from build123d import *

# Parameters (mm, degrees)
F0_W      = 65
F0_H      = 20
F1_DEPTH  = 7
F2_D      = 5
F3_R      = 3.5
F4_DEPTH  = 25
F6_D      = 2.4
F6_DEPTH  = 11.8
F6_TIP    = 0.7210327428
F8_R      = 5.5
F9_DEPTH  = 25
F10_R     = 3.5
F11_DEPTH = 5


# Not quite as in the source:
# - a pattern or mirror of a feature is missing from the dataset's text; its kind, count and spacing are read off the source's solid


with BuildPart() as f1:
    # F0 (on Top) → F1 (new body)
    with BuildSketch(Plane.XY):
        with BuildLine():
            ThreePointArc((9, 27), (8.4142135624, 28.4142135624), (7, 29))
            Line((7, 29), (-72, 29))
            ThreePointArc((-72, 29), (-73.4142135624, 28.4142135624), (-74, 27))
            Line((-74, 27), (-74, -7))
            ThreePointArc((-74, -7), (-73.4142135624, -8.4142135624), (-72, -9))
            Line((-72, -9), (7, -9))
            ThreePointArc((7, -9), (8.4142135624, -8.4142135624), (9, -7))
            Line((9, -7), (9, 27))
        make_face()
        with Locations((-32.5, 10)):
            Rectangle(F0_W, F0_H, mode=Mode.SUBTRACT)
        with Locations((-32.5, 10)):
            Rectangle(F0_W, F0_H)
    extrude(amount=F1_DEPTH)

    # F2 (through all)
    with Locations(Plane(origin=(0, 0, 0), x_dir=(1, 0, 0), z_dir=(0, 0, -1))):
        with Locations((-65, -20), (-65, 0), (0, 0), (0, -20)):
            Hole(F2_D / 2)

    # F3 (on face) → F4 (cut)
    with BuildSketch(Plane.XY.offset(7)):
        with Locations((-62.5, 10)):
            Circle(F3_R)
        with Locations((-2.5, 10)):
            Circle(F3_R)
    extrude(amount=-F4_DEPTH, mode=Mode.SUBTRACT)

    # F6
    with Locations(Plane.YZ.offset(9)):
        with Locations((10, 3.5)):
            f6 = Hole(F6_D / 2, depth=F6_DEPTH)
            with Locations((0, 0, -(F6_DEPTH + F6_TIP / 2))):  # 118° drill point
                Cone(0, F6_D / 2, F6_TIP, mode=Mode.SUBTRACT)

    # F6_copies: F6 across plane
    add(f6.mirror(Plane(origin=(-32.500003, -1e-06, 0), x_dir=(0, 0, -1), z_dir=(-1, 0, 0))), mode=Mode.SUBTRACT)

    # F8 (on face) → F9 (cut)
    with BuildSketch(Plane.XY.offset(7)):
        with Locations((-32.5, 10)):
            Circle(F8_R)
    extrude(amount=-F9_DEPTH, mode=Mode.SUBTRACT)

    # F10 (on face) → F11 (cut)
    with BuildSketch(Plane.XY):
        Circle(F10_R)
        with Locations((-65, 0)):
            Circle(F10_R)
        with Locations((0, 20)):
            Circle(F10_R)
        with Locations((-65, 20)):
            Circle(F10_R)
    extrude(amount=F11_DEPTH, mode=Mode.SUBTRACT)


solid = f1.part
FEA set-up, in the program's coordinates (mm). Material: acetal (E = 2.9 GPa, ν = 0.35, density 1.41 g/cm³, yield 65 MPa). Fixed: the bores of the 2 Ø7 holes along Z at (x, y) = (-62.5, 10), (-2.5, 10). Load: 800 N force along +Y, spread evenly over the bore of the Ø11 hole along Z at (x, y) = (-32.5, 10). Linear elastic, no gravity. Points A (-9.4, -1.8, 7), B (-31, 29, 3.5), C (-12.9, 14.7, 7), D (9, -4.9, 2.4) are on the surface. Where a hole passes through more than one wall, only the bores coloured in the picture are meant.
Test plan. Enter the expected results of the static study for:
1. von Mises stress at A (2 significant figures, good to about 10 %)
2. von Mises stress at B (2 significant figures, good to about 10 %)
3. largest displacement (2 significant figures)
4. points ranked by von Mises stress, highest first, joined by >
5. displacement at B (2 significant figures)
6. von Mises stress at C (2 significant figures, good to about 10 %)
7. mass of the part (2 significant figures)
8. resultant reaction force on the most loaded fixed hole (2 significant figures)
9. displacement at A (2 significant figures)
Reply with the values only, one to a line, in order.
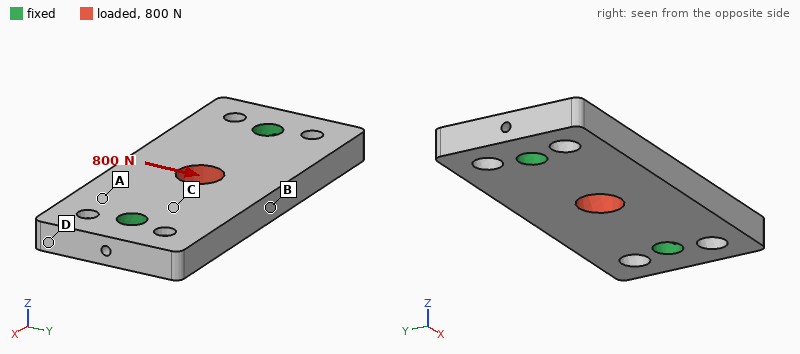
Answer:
2.2 MPa
6.5 MPa
76 µm
B > C > A > D
64 µm
3.6 MPa
28 g
400 N
25 µm
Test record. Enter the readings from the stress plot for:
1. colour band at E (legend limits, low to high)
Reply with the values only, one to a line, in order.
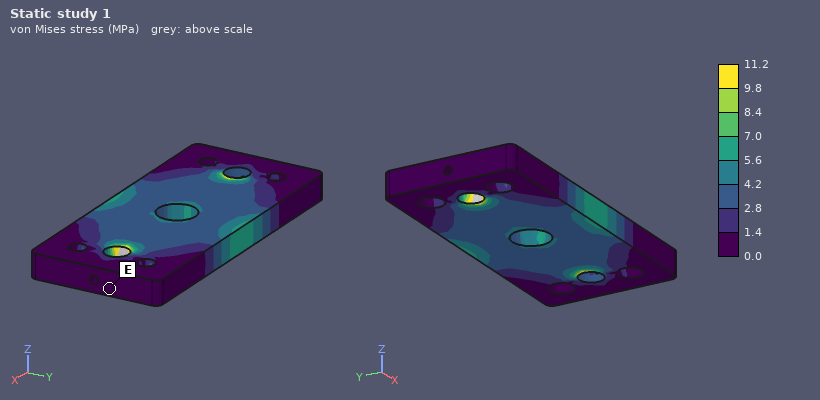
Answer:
0.0 to 1.4 MPa
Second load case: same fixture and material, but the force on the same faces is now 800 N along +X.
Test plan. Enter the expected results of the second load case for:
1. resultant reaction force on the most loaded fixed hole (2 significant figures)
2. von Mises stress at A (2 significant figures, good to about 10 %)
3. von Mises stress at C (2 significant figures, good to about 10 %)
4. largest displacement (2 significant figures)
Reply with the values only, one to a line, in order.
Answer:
400 N
0.69 MPa
2.9 MPa
28 µm
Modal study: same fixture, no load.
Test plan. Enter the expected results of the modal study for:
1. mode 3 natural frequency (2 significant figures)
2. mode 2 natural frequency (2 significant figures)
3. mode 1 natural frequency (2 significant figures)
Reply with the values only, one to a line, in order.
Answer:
4100 Hz
2400 Hz
2400 Hz
